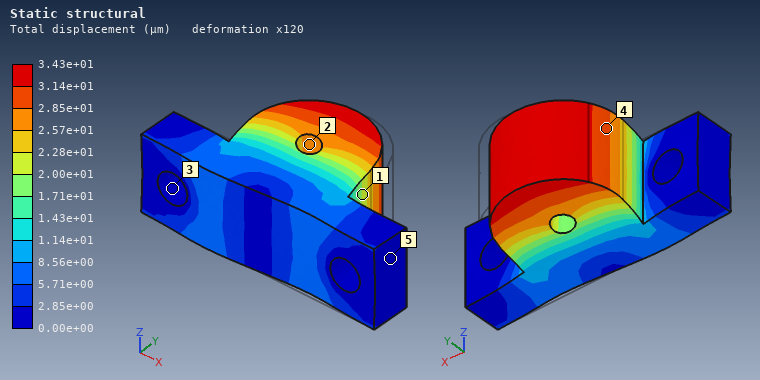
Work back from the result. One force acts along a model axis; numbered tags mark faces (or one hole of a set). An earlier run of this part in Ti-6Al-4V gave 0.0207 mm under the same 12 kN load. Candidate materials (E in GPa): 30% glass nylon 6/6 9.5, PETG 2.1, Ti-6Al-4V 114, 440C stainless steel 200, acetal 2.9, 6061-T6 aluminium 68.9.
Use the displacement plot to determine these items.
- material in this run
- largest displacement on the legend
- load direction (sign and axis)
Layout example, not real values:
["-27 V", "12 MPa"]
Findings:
["6061-T6 aluminium", "3.43e+01 µm", "-X"]
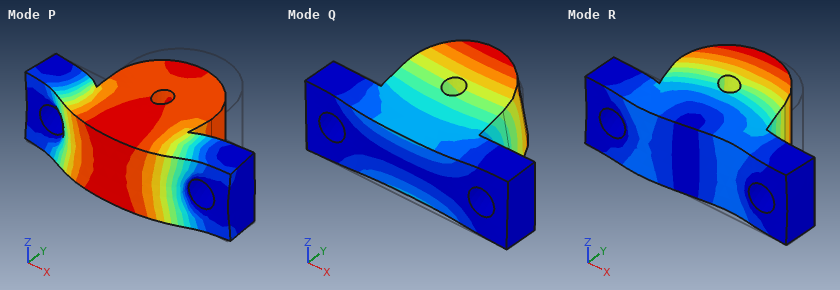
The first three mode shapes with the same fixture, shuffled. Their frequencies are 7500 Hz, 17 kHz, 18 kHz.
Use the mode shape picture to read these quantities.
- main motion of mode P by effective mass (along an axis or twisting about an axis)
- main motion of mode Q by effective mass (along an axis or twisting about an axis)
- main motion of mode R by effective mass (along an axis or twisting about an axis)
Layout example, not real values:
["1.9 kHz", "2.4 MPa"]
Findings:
["along Y", "along Z", "along X"]
